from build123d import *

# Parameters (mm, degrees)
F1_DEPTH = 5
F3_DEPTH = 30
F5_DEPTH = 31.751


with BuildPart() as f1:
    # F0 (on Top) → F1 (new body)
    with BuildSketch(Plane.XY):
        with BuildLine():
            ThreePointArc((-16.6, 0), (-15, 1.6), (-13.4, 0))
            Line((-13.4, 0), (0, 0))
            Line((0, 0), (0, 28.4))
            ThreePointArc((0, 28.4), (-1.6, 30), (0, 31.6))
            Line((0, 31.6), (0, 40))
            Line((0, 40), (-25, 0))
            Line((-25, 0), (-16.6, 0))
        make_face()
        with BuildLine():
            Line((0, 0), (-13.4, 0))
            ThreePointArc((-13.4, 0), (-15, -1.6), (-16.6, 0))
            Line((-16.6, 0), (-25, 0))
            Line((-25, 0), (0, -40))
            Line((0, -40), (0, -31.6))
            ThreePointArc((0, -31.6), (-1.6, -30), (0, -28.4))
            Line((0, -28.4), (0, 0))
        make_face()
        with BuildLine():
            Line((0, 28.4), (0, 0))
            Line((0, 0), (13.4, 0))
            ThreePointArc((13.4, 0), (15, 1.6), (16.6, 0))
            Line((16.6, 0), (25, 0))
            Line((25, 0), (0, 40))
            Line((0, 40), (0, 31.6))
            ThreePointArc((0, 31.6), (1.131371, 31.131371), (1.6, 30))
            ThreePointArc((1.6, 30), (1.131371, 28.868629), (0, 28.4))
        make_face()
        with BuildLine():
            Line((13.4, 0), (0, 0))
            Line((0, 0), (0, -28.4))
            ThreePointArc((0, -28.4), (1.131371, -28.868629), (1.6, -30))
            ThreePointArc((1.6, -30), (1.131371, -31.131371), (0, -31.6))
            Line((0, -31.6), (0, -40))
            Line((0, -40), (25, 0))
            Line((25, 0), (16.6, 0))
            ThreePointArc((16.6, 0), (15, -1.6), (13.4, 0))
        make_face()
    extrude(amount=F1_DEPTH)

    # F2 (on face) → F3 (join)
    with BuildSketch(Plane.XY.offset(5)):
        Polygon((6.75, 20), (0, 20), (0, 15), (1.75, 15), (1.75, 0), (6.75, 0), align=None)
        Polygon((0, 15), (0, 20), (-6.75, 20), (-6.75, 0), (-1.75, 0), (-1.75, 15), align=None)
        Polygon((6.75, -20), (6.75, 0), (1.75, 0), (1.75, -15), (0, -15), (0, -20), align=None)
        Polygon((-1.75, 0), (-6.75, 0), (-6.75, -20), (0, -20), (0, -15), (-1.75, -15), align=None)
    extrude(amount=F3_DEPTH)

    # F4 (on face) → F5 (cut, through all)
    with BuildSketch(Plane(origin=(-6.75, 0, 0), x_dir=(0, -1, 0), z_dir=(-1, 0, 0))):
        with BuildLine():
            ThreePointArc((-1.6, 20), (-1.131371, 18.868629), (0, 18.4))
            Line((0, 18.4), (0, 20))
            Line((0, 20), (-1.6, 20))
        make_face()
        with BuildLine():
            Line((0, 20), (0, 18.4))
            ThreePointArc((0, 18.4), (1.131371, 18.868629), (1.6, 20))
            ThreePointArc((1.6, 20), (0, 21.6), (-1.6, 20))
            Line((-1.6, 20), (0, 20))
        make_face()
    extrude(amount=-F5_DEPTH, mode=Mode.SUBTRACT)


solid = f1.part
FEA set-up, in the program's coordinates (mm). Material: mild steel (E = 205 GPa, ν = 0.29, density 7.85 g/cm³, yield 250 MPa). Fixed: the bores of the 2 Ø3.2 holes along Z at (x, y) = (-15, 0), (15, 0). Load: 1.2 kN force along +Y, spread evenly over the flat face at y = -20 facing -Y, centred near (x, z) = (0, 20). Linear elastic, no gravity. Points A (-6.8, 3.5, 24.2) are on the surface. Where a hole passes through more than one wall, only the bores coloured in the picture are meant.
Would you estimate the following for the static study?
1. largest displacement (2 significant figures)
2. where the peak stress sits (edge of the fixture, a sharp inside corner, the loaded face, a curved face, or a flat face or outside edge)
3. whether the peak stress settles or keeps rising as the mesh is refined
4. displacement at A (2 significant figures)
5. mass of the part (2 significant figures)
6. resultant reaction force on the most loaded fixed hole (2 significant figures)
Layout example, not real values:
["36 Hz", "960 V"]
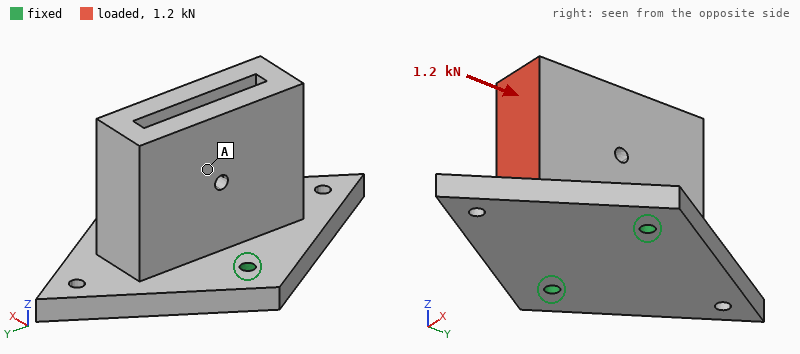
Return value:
["54 µm", "edge of the fixture", "keeps rising", "29 µm", "180 g", "600 N"]
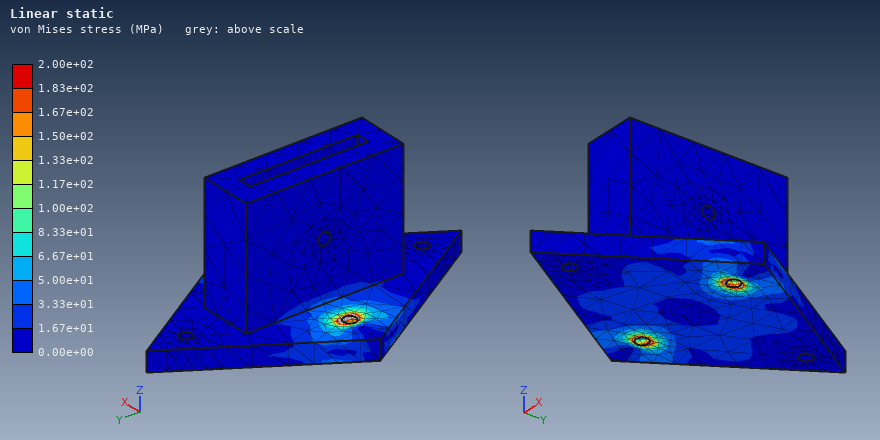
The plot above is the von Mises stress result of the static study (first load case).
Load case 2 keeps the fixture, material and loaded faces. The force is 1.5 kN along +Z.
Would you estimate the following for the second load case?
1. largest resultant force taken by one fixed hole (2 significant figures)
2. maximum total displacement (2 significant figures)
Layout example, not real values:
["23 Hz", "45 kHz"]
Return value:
["770 N", "81 µm"]
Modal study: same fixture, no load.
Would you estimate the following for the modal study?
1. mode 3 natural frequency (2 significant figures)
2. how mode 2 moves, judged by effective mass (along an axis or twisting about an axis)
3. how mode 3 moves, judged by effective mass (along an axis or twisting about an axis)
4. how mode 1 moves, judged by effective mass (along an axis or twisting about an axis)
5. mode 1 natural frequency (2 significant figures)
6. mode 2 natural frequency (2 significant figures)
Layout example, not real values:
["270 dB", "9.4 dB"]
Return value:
["7700 Hz", "along X", "along Z", "along Y", "2400 Hz", "5100 Hz"]
